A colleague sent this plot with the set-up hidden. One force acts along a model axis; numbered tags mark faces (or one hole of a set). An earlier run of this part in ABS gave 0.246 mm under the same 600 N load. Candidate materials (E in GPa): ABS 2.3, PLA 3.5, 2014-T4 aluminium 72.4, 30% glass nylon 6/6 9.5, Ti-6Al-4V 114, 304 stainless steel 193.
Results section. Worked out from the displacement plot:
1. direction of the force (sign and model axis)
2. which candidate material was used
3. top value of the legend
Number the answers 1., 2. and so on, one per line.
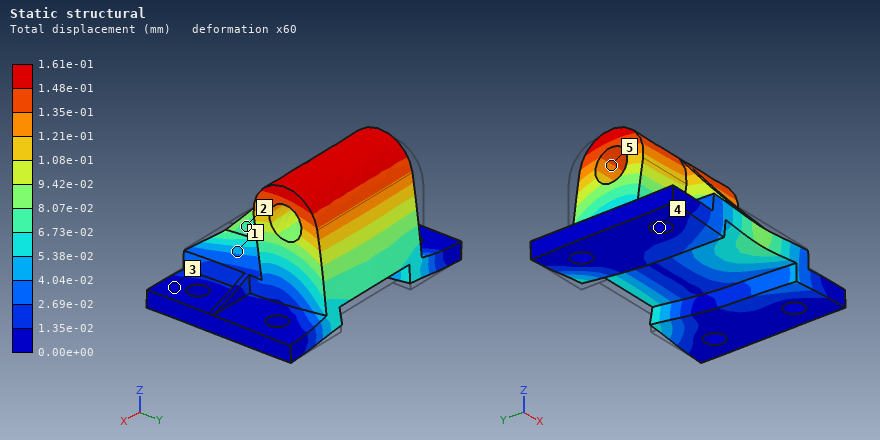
1. -Y
2. PLA
3. 1.61e-01 mm
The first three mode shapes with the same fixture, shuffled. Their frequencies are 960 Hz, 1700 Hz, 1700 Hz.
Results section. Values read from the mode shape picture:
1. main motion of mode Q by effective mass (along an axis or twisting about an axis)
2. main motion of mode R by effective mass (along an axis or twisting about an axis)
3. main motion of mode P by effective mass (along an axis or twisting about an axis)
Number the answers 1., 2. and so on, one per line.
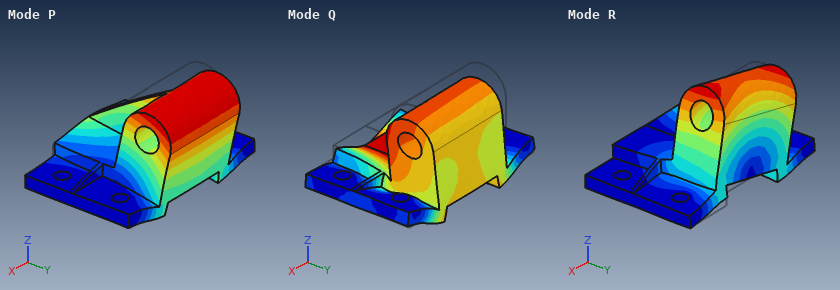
1. along Z
2. along X
3. along Y
